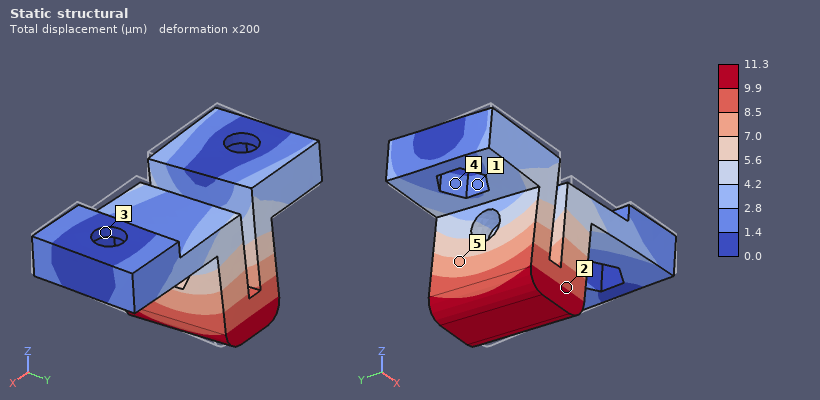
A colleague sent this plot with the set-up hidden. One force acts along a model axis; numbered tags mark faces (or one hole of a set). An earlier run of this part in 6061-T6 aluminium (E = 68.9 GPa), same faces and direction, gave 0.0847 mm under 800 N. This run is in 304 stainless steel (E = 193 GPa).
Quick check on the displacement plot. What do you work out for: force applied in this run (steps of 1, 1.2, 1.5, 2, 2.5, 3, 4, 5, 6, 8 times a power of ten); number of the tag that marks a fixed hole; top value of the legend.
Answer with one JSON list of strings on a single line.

["300 N", "3", "11.3 µm"]
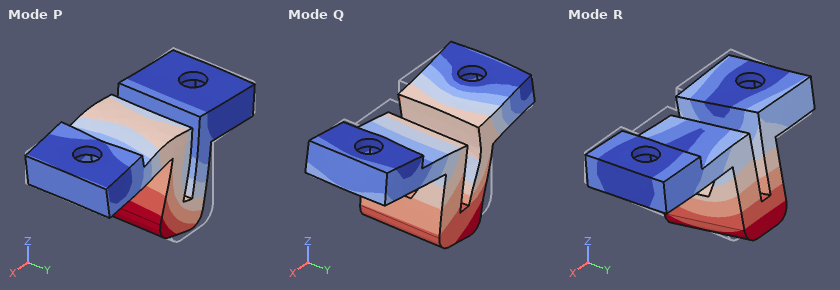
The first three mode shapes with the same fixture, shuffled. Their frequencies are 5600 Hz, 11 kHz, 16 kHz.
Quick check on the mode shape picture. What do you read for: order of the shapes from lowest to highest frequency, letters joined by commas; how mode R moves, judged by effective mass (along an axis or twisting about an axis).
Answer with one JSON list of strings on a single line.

["R, P, Q", "along Y"]
